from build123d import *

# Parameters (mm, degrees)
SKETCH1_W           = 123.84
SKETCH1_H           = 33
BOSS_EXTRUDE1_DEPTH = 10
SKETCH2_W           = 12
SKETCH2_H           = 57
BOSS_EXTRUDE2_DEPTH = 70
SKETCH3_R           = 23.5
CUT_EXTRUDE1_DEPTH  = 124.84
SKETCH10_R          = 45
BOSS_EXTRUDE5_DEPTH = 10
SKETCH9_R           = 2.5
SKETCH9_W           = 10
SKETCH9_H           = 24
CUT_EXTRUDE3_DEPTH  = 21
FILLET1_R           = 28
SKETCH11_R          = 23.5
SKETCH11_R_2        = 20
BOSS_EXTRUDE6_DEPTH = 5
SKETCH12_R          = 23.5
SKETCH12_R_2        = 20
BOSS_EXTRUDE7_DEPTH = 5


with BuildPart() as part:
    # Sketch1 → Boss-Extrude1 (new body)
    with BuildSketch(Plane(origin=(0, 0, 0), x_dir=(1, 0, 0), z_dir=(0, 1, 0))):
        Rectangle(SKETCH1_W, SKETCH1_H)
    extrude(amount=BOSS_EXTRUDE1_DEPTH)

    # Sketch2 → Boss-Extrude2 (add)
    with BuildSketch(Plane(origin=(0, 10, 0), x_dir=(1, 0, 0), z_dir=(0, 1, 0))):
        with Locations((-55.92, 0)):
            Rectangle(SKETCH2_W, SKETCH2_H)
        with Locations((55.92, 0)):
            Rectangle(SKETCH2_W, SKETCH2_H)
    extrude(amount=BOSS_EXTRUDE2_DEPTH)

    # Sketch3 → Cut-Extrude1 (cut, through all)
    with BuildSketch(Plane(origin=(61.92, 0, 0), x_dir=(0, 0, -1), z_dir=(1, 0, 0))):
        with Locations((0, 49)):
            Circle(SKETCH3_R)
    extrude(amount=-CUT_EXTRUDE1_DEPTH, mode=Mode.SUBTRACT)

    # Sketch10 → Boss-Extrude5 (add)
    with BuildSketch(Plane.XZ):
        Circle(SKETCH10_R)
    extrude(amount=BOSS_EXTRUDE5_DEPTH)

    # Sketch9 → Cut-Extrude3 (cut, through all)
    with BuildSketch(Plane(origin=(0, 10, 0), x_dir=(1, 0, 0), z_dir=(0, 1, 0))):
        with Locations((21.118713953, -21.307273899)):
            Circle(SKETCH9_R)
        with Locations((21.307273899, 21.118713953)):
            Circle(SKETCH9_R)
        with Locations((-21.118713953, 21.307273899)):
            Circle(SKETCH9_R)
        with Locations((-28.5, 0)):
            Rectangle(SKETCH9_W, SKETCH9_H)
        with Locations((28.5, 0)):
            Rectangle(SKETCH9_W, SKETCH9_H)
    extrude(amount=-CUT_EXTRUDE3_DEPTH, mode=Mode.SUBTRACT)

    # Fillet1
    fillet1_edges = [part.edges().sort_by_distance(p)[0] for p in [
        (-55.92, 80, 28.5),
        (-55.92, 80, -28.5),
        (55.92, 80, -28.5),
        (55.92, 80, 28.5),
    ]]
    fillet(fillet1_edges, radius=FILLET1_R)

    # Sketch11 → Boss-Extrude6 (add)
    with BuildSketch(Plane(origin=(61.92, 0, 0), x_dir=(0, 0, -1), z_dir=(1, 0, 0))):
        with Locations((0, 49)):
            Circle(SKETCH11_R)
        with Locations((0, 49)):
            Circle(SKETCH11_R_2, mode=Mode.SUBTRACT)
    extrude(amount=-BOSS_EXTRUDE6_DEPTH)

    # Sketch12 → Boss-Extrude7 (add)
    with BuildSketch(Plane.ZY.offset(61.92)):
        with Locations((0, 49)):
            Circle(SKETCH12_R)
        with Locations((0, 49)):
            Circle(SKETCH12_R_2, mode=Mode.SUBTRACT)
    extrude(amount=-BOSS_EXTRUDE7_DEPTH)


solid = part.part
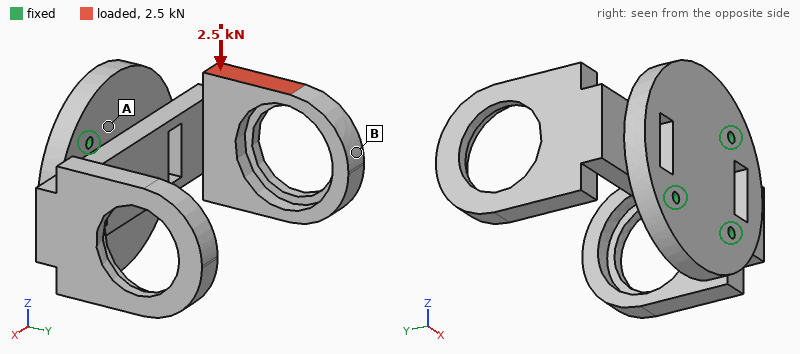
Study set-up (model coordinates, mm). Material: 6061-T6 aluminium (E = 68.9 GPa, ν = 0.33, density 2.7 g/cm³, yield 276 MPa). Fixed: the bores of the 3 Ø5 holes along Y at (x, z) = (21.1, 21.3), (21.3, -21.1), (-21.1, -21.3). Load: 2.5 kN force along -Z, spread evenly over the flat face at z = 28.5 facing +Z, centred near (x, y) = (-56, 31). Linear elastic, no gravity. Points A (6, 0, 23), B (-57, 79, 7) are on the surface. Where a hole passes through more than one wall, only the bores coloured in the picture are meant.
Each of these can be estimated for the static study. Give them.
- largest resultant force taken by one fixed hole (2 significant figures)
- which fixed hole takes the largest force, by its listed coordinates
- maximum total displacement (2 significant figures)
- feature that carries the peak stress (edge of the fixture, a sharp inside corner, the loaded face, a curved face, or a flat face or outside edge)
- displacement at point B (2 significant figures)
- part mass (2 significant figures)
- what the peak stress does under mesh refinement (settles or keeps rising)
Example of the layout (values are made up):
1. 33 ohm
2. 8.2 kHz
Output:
1. 3.5 kN
2. (21.1, 21.3)
3. 0.47 mm
4. edge of the fixture
5. 0.46 mm
6. 390 g
7. keeps rising
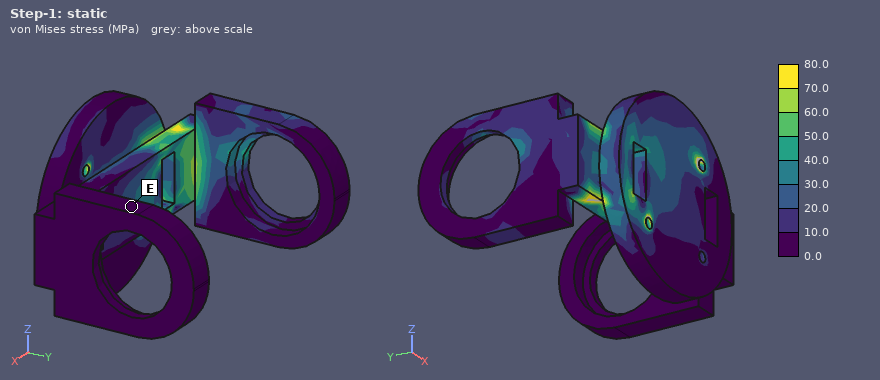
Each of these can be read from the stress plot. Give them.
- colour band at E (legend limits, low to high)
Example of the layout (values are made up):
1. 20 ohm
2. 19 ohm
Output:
1. 0.0 to 10.0 MPa
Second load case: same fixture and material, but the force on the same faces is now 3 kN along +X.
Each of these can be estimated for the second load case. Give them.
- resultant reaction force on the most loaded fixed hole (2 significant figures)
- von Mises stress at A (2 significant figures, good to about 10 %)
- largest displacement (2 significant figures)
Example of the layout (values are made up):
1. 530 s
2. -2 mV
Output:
1. 2.8 kN
2. 12 MPa
3. 1.1 mm
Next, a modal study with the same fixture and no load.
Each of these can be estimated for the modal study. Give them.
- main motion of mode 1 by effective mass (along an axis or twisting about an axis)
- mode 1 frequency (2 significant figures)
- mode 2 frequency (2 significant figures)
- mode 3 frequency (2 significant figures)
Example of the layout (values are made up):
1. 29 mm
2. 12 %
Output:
1. along X
2. 1000 Hz
3. 1100 Hz
4. 1500 Hz
